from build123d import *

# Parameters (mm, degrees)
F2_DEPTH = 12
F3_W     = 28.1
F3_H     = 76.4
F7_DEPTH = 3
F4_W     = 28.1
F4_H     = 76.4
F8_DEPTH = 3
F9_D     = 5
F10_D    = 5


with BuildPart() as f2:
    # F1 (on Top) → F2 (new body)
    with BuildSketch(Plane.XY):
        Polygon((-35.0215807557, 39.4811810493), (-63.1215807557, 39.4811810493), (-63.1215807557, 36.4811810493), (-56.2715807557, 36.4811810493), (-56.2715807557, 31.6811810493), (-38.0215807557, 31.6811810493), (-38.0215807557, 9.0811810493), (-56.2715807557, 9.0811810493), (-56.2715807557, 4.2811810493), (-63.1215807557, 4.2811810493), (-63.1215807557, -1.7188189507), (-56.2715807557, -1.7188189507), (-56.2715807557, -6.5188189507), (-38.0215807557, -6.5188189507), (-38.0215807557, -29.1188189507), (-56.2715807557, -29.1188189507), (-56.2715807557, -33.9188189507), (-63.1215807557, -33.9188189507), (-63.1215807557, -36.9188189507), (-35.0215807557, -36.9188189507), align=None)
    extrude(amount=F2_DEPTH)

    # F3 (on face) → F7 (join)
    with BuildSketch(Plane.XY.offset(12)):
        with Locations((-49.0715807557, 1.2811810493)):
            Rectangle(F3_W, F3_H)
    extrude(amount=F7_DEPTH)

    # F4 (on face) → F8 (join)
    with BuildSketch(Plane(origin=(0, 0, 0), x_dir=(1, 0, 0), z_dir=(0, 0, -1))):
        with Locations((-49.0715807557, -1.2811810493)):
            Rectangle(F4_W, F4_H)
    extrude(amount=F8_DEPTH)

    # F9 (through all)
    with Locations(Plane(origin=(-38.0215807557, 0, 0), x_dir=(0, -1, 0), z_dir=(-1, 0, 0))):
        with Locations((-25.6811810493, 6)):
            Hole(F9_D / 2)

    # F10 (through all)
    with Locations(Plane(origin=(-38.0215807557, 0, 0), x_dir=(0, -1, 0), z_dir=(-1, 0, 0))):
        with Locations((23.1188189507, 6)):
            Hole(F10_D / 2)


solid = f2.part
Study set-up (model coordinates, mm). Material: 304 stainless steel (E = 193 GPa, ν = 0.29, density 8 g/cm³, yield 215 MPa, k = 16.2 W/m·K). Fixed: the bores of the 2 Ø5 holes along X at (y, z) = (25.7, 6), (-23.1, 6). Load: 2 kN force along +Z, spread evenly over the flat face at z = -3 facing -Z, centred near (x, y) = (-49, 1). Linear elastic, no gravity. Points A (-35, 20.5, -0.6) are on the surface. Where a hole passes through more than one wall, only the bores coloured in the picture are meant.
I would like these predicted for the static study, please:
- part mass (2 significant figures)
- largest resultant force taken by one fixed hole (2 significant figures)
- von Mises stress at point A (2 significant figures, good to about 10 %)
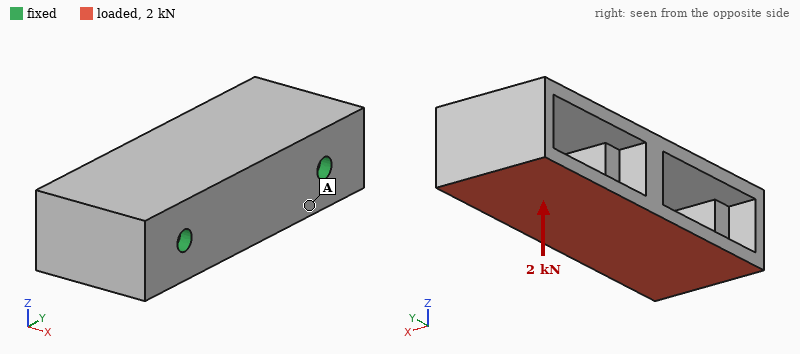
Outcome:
190 g
1.0 kN
35 MPa
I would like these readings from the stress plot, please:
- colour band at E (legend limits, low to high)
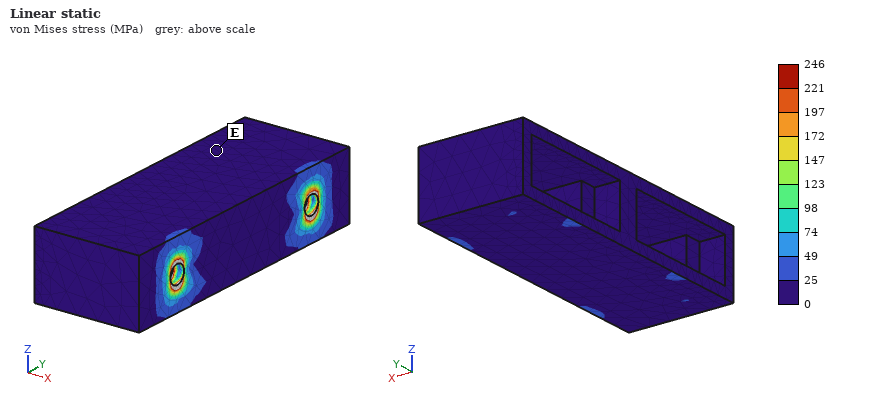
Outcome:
0 to 25 MPa
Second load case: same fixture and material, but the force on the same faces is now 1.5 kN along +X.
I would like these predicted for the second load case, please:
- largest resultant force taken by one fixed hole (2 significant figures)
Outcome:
760 N
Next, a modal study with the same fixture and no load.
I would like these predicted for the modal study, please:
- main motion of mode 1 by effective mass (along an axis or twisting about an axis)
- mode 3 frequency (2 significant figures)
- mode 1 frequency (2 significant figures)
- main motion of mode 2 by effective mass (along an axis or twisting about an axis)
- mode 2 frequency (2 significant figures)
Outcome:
along Z
7600 Hz
2800 Hz
twisting about X
6400 Hz
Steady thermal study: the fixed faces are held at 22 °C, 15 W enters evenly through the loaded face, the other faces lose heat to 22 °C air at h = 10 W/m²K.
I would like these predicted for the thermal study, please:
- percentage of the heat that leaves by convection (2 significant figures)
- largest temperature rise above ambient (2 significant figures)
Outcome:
21 %
54 K
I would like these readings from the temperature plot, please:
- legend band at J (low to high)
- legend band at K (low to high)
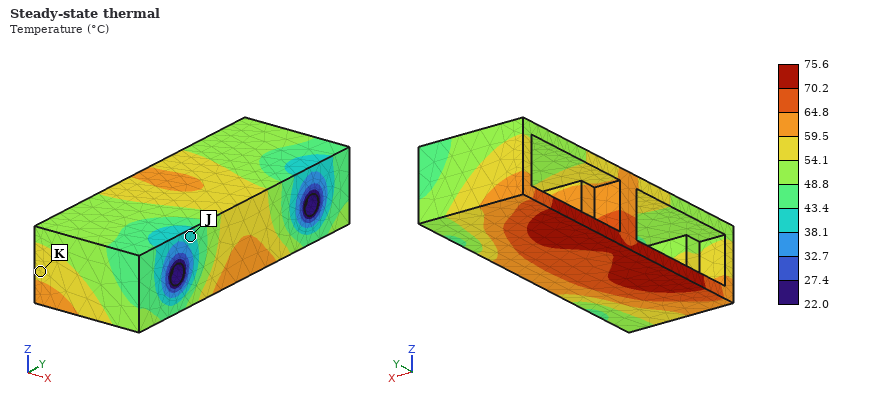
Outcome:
38.1 to 43.4 °C
54.1 to 59.5 °C
